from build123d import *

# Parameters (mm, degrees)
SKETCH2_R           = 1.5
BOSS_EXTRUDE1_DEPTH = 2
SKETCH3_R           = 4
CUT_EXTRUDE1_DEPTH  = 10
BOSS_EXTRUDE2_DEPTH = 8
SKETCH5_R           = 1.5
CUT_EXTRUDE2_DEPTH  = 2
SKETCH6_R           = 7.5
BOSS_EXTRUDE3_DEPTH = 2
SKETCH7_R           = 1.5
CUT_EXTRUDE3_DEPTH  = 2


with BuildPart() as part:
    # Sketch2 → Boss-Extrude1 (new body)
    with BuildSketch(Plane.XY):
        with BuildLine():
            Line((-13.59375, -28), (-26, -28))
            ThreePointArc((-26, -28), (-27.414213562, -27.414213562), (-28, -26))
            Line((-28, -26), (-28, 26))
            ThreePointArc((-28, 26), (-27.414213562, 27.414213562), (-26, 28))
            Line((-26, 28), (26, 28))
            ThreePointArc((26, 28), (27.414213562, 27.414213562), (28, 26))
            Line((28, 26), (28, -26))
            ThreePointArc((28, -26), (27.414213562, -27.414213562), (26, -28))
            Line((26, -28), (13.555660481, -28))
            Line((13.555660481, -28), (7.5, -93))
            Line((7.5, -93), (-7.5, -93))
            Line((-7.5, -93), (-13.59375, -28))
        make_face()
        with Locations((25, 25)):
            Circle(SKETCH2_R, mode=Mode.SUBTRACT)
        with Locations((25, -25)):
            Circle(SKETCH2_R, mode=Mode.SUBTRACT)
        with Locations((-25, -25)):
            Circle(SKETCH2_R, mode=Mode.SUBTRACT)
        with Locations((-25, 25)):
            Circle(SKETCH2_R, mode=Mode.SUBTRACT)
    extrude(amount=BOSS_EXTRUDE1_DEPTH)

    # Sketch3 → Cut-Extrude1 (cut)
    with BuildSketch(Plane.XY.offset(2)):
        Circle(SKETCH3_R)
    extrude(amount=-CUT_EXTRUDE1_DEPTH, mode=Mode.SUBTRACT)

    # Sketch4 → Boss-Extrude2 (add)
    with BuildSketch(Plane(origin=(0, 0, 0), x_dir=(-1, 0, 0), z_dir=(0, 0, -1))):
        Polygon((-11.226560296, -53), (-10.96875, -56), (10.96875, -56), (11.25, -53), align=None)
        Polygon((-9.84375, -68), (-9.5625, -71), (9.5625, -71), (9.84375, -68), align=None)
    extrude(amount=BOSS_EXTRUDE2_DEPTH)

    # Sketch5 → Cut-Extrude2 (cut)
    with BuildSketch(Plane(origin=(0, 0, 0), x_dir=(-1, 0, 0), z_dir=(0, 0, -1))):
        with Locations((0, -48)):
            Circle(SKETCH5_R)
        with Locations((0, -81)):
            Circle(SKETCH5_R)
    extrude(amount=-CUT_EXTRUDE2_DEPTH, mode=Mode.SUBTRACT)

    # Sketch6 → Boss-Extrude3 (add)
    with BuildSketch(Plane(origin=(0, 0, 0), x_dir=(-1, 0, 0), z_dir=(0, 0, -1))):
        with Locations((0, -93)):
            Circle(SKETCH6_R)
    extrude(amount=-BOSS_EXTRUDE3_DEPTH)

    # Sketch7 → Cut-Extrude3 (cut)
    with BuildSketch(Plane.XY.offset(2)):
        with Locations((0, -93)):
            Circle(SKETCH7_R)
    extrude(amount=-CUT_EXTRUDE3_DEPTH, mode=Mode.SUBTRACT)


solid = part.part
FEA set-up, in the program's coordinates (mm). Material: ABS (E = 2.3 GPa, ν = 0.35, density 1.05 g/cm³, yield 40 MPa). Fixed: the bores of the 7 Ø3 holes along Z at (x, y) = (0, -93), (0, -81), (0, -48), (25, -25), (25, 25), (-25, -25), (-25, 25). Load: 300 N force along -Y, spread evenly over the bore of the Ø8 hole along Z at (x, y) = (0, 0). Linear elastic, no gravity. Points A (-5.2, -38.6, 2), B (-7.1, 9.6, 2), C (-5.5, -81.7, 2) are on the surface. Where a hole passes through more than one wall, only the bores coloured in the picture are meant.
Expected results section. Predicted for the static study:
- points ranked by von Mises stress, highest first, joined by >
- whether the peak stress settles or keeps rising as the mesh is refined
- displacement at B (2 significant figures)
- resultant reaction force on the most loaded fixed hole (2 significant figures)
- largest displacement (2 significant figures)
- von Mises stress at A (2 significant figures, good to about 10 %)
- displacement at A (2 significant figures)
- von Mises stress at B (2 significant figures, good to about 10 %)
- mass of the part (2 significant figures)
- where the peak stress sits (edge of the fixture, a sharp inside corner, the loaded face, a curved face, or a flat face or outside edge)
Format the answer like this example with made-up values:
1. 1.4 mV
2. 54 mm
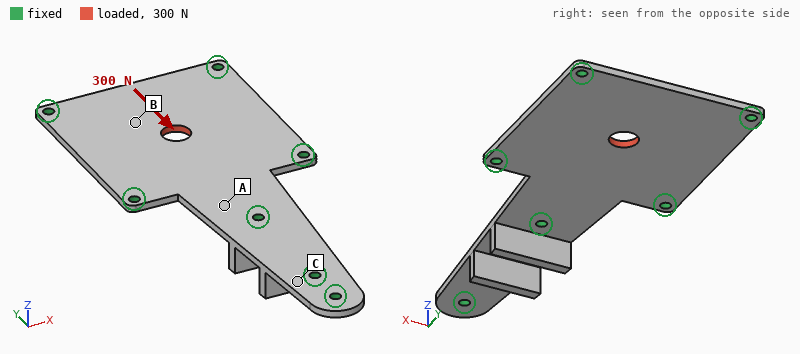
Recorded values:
1. B > A > C
2. keeps rising
3. 39 µm
4. 67 N
5. 59 µm
6. 1.7 MPa
7. 11 µm
8. 3.0 MPa
9. 10 g
10. edge of the fixture
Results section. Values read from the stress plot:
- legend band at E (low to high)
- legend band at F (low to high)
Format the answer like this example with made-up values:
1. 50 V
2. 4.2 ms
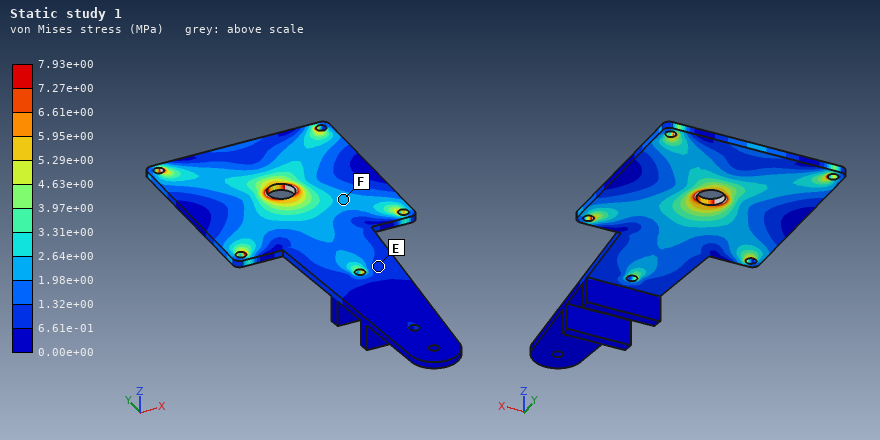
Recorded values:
1. 6.61e-01 to 1.32e+00 MPa
2. 1.98e+00 to 2.64e+00 MPa
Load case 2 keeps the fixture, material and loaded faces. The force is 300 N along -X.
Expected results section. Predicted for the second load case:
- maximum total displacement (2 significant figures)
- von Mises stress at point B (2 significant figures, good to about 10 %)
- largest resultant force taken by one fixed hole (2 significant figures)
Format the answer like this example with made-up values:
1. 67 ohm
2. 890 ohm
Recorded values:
1. 66 µm
2. 3.2 MPa
3. 85 N
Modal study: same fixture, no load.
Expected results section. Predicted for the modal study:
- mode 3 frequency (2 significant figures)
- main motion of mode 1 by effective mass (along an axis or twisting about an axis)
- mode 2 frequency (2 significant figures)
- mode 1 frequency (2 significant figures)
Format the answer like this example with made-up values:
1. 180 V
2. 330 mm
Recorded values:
1. 1400 Hz
2. along Z
3. 1400 Hz
4. 800 Hz
